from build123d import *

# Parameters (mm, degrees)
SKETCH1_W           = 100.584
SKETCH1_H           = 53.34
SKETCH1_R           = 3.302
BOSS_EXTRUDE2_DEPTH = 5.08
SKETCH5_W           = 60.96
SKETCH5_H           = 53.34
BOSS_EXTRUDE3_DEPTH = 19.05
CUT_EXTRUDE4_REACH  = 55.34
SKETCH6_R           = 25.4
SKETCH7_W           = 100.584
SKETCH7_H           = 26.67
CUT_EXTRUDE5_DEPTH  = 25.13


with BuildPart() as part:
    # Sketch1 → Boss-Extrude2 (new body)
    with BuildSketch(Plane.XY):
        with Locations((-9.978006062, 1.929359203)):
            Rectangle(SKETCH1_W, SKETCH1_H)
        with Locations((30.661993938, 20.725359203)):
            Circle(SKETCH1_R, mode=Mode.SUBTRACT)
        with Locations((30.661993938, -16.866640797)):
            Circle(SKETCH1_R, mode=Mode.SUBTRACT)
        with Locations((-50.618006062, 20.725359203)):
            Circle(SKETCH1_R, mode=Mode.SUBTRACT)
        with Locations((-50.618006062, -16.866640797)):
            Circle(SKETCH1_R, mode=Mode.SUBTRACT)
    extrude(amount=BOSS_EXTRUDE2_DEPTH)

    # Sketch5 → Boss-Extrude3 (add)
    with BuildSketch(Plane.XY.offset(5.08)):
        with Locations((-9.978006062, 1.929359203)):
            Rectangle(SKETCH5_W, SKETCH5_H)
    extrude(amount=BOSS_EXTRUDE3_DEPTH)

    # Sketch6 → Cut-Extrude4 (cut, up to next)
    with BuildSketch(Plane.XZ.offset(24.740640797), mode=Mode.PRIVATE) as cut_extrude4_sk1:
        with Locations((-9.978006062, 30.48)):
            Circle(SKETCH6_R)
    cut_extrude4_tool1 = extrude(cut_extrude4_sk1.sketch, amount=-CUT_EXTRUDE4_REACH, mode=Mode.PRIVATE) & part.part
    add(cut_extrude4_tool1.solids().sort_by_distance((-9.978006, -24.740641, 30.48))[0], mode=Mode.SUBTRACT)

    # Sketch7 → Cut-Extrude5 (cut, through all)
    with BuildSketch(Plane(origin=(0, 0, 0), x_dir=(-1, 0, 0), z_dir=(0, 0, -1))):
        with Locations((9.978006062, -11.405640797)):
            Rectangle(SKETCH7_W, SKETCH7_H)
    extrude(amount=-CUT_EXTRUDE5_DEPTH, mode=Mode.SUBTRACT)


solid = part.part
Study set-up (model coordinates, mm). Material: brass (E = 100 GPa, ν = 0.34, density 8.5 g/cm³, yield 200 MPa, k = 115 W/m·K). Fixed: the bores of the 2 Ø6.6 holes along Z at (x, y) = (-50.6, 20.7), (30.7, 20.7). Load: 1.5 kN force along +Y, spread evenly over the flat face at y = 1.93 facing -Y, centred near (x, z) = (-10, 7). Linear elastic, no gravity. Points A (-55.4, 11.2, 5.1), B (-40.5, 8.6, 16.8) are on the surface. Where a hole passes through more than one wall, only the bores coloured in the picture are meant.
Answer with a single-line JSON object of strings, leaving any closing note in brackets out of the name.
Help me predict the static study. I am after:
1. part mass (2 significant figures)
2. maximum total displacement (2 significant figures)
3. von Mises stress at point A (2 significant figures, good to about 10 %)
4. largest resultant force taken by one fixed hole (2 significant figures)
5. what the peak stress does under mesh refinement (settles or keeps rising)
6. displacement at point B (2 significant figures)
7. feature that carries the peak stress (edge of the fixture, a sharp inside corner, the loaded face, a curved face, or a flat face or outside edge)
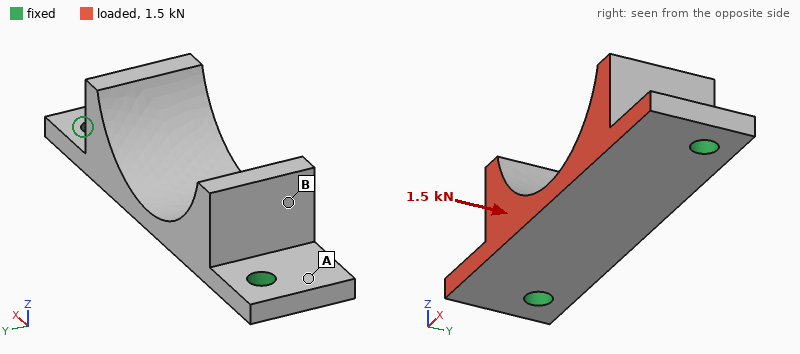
{"part mass": "220 g", "maximum total displacement": "25 µm", "von Mises stress at point A": "10 MPa", "largest resultant force taken by one fixed hole": "810 N", "what the peak stress does under mesh refinement": "keeps rising", "displacement at point B": "16 µm", "feature that carries the peak stress": "edge of the fixture"}
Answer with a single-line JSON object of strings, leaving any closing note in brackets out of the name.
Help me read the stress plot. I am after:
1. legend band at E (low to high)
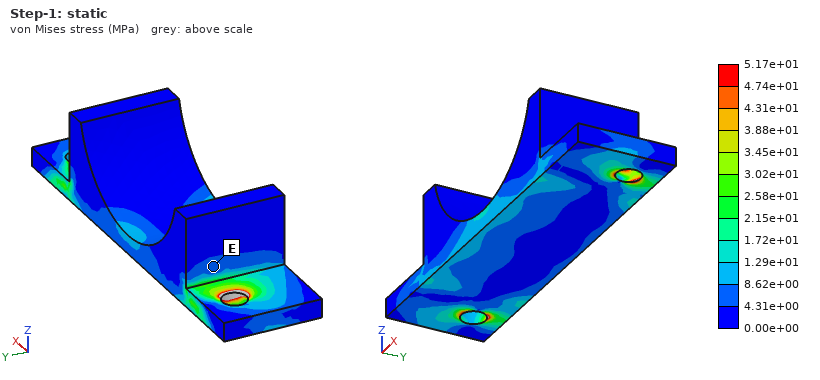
{"legend band at E": "4.31e+00 to 8.62e+00 MPa"}
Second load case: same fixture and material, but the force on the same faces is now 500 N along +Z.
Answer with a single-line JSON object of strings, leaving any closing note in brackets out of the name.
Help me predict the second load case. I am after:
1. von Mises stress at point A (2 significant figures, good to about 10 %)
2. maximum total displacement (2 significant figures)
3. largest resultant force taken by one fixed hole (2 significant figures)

{"von Mises stress at point A": "16 MPa", "maximum total displacement": "35 µm", "largest resultant force taken by one fixed hole": "270 N"}
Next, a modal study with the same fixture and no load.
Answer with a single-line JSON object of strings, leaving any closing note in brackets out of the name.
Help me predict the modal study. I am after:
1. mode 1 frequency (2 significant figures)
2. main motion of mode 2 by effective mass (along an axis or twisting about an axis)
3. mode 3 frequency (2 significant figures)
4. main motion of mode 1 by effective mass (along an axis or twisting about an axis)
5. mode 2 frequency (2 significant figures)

{"mode 1 frequency": "2000 Hz", "main motion of mode 2 by effective mass": "along Y", "mode 3 frequency": "4500 Hz", "main motion of mode 1 by effective mass": "along Z", "mode 2 frequency": "3100 Hz"}
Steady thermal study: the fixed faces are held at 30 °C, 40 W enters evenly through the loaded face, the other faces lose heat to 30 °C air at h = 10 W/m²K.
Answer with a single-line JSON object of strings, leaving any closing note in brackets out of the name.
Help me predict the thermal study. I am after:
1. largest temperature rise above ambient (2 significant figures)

{"largest temperature rise above ambient": "24 K"}
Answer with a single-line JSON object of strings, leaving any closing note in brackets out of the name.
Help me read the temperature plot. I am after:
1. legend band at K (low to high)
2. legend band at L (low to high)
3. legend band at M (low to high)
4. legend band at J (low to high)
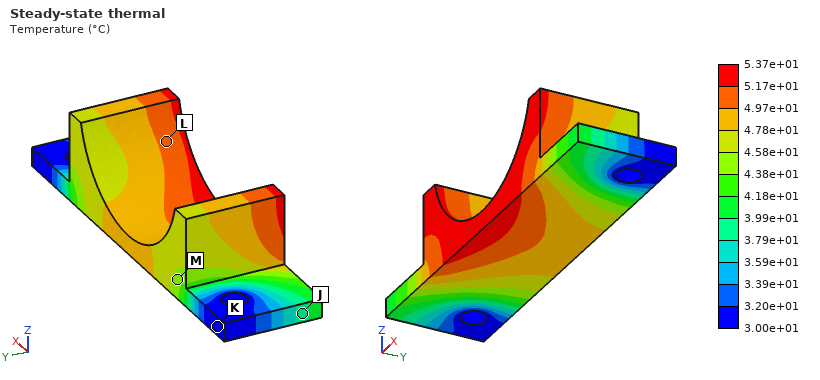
{"legend band at K": "3.00e+01 to 3.20e+01 °C", "legend band at L": "4.97e+01 to 5.17e+01 °C", "legend band at M": "4.38e+01 to 4.58e+01 °C", "legend band at J": "3.79e+01 to 3.99e+01 °C"}
